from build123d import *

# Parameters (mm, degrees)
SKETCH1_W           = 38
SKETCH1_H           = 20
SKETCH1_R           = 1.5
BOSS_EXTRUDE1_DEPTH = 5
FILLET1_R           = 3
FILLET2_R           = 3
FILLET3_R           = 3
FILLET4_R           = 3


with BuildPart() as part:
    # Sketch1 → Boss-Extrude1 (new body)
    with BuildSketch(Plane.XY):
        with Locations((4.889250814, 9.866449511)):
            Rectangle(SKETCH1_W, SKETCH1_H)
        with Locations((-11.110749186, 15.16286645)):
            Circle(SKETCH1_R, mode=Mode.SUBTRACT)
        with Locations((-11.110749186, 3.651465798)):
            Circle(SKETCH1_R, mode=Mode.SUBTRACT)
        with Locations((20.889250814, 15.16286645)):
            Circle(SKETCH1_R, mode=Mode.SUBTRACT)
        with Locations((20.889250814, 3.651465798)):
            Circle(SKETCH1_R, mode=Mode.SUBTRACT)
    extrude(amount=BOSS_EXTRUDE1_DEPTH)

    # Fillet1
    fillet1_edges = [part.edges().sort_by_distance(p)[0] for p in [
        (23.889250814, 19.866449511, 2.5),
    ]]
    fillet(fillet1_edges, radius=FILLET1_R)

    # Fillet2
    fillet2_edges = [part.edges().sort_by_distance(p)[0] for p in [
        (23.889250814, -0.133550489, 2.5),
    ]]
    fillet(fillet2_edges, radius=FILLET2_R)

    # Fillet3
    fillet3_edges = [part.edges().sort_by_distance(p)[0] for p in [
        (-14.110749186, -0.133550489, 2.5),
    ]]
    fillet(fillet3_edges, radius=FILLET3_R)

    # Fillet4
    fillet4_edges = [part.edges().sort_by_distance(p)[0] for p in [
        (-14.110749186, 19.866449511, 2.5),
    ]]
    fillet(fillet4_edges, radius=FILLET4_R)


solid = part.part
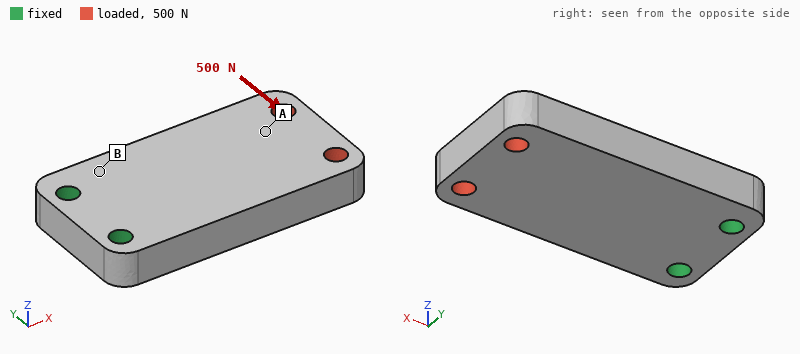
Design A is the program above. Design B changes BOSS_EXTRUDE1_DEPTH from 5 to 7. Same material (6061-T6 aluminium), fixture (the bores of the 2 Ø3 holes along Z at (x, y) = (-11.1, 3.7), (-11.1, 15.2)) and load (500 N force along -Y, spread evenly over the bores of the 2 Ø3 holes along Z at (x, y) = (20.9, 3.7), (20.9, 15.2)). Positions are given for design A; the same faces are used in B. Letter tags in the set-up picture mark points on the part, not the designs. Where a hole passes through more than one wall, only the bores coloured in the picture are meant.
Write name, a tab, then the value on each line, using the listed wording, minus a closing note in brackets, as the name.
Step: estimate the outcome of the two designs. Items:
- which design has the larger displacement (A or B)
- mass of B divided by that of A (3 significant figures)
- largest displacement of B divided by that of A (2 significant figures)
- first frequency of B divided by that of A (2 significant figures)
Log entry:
which design has the larger displacement	A
mass of B divided by that of A	1.40
largest displacement of B divided by that of A	0.71
first frequency of B divided by that of A	1.4
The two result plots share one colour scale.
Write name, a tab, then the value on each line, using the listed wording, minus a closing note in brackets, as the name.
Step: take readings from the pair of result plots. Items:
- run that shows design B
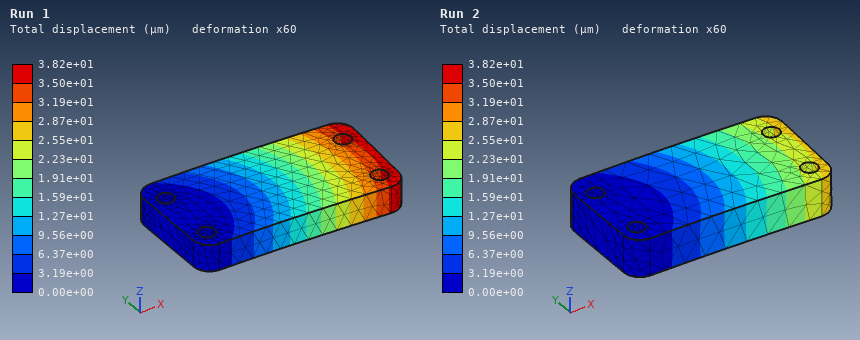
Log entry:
run that shows design B	Run 2
